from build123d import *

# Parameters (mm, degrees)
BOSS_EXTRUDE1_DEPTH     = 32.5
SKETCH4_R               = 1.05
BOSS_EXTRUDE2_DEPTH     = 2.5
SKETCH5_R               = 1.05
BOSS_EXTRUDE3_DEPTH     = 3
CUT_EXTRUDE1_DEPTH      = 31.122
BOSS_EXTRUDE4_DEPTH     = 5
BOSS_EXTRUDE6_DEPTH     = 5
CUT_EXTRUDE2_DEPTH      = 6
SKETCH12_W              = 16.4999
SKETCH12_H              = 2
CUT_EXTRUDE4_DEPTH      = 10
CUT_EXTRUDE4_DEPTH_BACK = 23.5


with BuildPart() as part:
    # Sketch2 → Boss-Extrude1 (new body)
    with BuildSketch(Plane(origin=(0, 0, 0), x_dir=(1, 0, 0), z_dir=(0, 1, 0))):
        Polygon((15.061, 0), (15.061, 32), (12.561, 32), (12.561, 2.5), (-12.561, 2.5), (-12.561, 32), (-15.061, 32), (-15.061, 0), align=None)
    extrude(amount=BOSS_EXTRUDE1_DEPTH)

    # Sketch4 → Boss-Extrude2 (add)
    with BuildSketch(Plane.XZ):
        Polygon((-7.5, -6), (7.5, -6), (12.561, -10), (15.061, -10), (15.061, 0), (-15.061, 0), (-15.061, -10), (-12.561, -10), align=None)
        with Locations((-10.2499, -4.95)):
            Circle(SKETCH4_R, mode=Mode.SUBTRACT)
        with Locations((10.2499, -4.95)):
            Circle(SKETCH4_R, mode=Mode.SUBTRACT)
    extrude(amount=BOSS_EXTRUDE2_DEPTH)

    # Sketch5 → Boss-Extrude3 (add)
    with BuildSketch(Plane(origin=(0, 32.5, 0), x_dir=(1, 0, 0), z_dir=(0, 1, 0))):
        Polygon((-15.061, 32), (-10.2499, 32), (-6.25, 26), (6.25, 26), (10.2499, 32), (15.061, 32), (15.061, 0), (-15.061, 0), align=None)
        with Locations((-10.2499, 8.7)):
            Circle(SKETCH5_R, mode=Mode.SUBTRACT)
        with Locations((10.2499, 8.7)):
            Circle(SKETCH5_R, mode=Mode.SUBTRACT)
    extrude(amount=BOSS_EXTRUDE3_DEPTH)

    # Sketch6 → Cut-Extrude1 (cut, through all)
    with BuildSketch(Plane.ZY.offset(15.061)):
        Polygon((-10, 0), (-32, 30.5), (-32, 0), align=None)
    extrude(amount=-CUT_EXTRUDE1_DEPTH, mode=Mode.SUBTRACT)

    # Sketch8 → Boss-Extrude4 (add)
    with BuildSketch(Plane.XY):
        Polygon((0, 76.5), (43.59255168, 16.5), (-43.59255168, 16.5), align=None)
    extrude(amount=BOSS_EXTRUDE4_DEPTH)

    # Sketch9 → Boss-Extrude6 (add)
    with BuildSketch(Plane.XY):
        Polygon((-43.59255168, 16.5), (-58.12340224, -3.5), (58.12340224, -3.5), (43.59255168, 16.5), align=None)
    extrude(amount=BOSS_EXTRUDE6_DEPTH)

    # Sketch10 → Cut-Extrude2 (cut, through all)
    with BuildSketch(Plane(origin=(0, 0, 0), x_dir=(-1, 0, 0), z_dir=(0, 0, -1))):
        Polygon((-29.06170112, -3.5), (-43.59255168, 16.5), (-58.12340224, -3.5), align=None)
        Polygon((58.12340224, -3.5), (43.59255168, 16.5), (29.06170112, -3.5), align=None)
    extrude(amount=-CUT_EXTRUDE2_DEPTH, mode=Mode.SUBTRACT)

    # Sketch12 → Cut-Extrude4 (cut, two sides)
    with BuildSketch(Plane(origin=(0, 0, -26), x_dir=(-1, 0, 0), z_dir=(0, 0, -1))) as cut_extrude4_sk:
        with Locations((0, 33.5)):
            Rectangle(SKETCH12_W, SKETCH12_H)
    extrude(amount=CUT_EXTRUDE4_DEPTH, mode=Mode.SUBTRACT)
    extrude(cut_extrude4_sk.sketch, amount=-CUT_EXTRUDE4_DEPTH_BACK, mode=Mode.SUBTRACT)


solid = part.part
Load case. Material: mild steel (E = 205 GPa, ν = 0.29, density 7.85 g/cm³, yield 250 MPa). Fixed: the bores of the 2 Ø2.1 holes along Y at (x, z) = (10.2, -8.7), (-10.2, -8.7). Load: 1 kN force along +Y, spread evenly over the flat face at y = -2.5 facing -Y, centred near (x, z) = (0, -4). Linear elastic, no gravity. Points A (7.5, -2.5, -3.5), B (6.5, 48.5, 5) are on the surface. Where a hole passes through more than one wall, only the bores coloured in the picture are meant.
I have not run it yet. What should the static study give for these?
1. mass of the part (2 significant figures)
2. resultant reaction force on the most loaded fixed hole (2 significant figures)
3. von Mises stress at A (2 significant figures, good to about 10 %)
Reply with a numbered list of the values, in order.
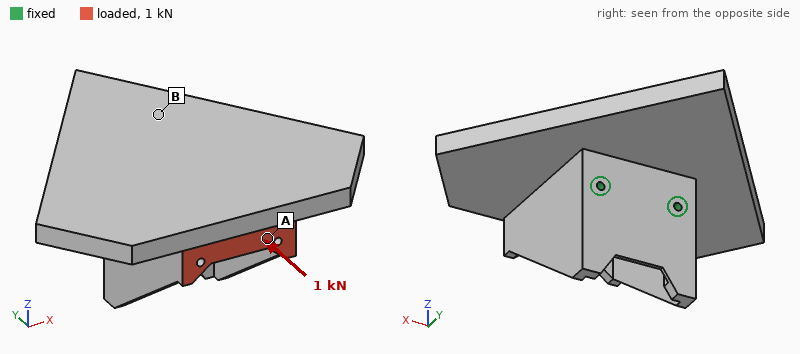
1. 220 g
2. 500 N
3. 14 MPa
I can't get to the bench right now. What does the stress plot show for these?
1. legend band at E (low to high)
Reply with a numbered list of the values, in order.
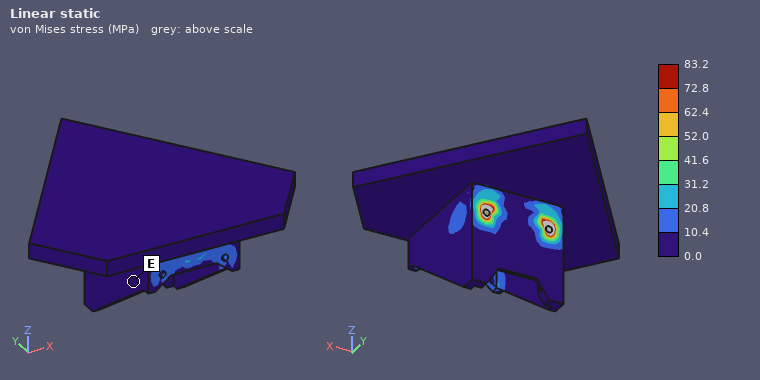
1. 0.0 to 10.4 MPa
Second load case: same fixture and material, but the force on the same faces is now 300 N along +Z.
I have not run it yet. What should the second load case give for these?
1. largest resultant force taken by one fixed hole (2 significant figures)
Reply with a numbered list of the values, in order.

1. 160 N
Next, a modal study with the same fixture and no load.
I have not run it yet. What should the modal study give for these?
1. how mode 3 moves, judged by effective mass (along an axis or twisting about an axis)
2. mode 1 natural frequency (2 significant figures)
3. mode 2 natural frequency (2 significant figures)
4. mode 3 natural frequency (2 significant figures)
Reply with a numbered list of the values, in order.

1. along X
2. 1000 Hz
3. 2500 Hz
4. 3900 Hz
